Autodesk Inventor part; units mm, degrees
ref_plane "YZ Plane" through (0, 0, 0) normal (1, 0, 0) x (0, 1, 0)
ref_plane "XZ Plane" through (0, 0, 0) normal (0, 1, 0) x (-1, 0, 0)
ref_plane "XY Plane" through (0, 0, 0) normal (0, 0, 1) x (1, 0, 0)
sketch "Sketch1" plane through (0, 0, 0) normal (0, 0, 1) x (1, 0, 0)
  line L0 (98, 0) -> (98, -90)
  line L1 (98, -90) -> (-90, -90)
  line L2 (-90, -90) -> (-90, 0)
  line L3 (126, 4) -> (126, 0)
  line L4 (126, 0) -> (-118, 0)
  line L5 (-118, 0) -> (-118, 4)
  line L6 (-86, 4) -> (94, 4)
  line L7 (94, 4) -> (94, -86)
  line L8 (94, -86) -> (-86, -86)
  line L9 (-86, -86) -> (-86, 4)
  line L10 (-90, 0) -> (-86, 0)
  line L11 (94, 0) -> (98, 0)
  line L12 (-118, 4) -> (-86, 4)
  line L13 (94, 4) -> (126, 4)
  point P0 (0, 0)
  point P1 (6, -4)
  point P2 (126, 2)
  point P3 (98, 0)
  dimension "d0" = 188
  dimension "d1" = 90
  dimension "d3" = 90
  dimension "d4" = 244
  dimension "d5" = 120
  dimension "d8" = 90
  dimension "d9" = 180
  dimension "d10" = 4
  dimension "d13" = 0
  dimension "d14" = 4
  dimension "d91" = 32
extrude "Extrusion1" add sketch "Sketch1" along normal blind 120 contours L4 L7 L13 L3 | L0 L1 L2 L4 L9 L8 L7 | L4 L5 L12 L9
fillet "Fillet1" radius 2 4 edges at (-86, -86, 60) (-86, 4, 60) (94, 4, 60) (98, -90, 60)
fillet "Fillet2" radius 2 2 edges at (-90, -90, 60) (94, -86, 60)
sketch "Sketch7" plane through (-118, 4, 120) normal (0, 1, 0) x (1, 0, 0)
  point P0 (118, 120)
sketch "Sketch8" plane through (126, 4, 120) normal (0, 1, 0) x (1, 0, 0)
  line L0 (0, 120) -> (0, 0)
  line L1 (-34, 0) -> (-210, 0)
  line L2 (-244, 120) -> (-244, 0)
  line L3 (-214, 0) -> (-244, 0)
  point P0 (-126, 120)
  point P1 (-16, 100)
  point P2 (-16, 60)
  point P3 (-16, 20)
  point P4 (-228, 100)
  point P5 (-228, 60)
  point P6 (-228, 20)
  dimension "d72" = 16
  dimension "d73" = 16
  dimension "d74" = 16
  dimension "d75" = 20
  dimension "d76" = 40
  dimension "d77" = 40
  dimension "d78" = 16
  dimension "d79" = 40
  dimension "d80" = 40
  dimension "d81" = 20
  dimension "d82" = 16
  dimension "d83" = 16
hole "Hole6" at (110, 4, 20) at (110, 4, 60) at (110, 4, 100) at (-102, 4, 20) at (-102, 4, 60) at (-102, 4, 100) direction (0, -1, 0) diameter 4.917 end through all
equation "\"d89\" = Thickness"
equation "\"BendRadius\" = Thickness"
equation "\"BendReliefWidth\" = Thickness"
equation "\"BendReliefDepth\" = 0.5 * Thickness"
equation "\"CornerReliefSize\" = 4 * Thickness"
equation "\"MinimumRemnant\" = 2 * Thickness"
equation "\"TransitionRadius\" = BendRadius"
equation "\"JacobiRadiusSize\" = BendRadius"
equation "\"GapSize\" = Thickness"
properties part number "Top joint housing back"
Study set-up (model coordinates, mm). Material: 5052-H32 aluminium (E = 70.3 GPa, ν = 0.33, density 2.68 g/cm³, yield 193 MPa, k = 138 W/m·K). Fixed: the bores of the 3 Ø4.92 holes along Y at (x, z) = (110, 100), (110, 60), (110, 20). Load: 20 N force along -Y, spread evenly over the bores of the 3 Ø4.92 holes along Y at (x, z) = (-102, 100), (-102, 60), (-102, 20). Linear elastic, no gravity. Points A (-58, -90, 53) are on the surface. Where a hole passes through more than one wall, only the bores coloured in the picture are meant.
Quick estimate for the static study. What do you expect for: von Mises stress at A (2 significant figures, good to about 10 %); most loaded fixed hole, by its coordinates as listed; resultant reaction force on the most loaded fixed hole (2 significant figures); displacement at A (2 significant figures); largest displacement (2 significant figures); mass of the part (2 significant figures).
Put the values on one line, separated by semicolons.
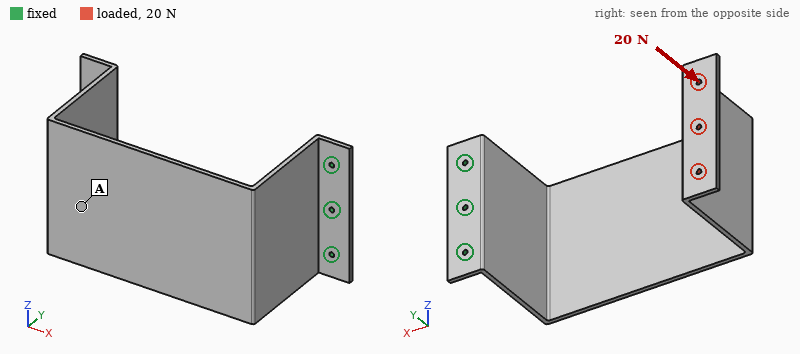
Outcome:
2.6 MPa; (110, 60); 21 N; 2.1 mm; 3.2 mm; 540 g
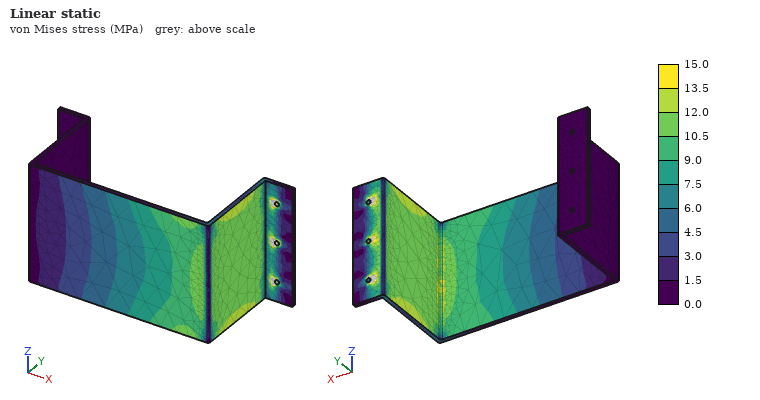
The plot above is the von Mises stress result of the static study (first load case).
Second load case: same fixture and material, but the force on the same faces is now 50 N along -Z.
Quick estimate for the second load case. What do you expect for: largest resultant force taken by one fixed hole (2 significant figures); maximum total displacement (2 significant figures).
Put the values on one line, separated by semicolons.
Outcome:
130 N; 3.2 mm
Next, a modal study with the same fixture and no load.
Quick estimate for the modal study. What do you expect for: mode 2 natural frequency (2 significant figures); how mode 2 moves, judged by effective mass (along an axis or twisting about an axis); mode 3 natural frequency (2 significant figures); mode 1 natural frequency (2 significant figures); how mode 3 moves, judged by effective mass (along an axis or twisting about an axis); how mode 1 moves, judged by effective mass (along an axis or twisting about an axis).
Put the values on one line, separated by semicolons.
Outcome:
54 Hz; along Z; 97 Hz; 30 Hz; along X; along Y
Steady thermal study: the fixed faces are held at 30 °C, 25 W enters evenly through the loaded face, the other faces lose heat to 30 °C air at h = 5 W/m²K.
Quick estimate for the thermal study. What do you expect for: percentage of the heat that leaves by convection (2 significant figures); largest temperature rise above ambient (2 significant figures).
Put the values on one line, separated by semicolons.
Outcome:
67 %; 79 K
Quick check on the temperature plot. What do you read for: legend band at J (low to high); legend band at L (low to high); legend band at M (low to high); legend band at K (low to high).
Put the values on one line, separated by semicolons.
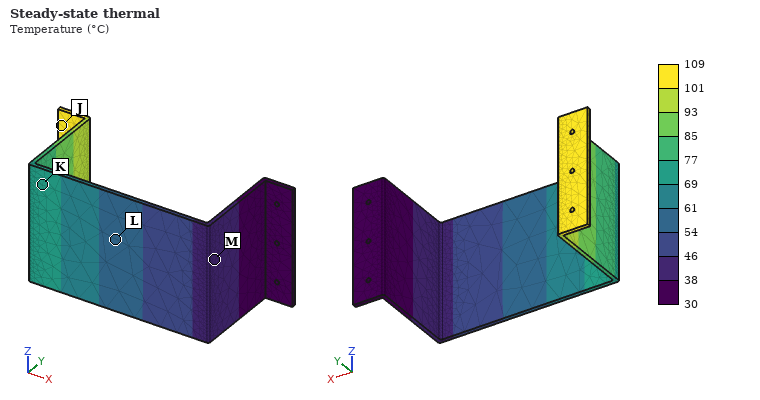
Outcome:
101 to 109 °C; 54 to 61 °C; 38 to 46 °C; 69 to 77 °C
